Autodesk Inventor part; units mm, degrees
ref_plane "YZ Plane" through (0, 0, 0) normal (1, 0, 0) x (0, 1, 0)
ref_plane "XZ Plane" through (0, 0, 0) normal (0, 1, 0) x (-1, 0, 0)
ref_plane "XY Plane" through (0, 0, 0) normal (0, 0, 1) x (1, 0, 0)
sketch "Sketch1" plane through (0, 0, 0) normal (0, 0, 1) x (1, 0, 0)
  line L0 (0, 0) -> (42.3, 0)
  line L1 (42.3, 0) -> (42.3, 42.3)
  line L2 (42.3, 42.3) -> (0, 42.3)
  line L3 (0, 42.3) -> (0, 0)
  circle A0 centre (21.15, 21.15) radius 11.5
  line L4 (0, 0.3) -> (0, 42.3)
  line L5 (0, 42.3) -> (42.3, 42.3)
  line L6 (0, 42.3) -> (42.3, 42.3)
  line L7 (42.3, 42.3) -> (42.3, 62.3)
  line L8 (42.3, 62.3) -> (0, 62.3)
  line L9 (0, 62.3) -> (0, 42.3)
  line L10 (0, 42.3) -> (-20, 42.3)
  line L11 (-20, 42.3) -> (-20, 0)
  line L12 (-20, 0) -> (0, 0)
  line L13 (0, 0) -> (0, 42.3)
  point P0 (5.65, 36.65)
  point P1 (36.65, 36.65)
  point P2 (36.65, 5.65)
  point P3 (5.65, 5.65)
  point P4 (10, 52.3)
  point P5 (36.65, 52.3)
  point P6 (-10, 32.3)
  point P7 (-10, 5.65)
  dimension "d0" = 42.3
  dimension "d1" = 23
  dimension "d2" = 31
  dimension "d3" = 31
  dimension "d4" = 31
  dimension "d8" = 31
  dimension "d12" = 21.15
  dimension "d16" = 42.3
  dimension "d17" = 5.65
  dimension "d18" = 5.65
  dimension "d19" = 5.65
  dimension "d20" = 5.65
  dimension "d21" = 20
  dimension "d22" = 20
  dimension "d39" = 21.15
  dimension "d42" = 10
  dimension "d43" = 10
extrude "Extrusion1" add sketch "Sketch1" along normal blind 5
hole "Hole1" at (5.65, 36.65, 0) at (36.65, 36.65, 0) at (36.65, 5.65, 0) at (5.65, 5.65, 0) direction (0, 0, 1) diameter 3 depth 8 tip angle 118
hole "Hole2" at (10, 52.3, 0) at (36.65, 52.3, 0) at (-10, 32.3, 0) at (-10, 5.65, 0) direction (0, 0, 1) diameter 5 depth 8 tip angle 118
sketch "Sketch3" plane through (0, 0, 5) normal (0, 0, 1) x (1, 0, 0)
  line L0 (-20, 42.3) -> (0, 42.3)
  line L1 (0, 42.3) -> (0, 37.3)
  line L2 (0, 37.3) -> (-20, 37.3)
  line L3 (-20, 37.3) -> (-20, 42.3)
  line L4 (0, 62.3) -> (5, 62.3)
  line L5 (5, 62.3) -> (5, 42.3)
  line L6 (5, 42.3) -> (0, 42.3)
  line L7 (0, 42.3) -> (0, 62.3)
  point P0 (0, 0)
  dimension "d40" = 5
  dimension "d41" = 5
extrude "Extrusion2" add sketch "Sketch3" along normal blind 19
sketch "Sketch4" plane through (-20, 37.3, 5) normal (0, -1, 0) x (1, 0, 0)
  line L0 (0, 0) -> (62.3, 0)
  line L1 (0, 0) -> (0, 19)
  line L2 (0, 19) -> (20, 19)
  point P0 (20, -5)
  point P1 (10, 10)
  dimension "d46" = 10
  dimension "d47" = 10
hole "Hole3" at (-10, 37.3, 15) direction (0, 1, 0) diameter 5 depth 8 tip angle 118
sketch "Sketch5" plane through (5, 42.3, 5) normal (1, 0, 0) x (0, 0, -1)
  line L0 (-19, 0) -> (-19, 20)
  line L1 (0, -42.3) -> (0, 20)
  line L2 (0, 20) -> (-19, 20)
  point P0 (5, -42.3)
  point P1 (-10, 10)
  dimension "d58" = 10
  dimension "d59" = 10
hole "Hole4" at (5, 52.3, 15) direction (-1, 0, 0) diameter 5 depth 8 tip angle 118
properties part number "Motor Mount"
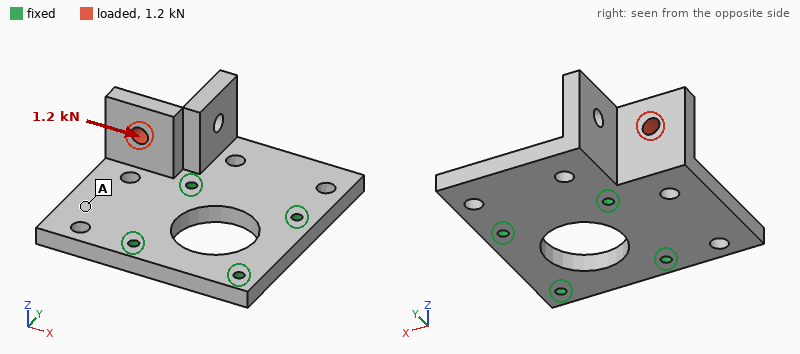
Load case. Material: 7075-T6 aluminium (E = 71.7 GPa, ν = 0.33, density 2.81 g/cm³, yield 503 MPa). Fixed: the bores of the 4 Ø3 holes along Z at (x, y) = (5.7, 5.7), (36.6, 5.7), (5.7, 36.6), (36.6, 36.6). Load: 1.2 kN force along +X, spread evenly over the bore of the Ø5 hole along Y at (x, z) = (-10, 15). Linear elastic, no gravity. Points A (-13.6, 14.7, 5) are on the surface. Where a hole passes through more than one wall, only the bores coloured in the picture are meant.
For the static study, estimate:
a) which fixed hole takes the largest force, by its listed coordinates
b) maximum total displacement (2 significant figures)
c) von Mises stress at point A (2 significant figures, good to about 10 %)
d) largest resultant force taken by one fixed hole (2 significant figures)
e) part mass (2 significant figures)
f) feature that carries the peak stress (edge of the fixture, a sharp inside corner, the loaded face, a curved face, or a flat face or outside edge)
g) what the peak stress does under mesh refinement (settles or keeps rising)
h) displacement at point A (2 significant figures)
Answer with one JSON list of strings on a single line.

["(5.7, 36.6)", "0.20 mm", "21 MPa", "1.0 kN", "52 g", "edge of the fixture", "keeps rising", "0.042 mm"]
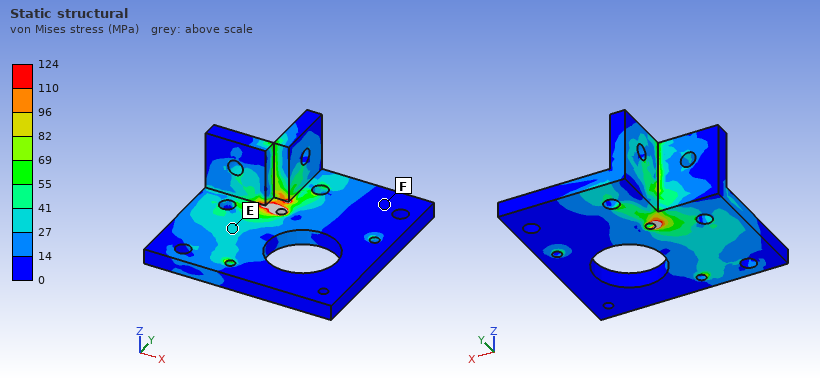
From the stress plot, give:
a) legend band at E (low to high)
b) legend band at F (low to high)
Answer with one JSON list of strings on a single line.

["27 to 41 MPa", "0 to 14 MPa"]
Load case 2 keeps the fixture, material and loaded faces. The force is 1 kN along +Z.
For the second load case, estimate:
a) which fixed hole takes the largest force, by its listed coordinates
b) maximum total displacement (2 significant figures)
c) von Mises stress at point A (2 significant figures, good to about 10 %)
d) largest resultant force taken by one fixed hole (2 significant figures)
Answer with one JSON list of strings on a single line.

["(5.7, 36.6)", "0.17 mm", "20 MPa", "1.2 kN"]
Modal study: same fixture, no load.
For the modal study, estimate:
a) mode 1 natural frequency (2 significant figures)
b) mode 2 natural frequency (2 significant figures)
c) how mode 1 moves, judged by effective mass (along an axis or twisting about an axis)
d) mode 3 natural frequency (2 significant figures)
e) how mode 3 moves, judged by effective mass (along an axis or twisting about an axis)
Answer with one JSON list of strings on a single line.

["3900 Hz", "4200 Hz", "along Z", "7100 Hz", "along Z"]
